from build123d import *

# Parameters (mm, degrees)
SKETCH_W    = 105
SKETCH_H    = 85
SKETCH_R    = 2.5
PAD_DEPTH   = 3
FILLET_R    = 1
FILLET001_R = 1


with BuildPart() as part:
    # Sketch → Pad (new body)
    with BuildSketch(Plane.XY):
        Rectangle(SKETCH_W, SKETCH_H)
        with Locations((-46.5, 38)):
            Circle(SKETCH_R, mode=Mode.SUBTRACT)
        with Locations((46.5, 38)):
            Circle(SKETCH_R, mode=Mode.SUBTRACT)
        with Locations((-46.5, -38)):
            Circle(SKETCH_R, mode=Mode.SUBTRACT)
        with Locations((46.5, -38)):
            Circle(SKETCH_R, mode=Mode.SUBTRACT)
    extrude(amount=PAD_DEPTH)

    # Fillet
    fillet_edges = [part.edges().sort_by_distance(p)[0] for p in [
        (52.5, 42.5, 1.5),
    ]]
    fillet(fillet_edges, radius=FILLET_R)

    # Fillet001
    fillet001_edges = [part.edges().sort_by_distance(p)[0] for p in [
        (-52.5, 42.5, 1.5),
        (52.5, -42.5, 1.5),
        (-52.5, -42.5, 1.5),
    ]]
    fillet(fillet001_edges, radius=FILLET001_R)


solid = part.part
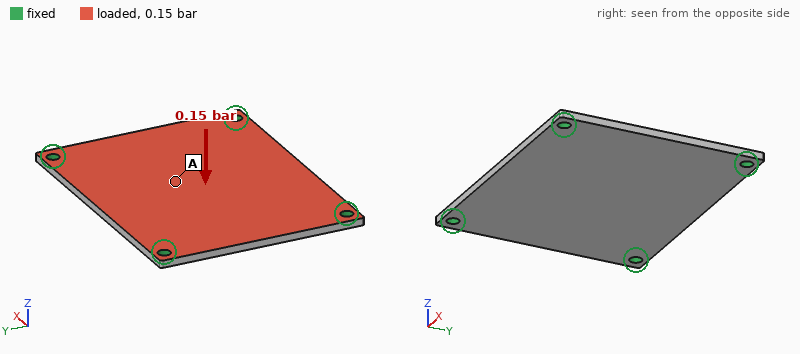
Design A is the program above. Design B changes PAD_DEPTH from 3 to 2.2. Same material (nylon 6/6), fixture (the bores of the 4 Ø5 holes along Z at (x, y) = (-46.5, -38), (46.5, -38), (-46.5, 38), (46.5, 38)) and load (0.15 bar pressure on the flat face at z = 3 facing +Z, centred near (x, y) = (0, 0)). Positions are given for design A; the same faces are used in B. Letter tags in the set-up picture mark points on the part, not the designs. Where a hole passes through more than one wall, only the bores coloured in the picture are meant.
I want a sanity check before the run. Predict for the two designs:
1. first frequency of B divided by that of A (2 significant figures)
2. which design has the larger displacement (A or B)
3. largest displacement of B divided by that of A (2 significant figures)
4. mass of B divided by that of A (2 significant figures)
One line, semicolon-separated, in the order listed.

0.75; B; 2.5; 0.73
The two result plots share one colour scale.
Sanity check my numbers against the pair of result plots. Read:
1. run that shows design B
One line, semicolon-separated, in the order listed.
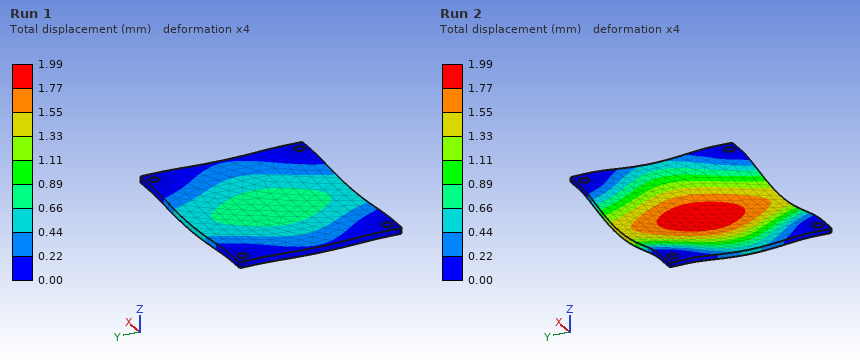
Run 2
